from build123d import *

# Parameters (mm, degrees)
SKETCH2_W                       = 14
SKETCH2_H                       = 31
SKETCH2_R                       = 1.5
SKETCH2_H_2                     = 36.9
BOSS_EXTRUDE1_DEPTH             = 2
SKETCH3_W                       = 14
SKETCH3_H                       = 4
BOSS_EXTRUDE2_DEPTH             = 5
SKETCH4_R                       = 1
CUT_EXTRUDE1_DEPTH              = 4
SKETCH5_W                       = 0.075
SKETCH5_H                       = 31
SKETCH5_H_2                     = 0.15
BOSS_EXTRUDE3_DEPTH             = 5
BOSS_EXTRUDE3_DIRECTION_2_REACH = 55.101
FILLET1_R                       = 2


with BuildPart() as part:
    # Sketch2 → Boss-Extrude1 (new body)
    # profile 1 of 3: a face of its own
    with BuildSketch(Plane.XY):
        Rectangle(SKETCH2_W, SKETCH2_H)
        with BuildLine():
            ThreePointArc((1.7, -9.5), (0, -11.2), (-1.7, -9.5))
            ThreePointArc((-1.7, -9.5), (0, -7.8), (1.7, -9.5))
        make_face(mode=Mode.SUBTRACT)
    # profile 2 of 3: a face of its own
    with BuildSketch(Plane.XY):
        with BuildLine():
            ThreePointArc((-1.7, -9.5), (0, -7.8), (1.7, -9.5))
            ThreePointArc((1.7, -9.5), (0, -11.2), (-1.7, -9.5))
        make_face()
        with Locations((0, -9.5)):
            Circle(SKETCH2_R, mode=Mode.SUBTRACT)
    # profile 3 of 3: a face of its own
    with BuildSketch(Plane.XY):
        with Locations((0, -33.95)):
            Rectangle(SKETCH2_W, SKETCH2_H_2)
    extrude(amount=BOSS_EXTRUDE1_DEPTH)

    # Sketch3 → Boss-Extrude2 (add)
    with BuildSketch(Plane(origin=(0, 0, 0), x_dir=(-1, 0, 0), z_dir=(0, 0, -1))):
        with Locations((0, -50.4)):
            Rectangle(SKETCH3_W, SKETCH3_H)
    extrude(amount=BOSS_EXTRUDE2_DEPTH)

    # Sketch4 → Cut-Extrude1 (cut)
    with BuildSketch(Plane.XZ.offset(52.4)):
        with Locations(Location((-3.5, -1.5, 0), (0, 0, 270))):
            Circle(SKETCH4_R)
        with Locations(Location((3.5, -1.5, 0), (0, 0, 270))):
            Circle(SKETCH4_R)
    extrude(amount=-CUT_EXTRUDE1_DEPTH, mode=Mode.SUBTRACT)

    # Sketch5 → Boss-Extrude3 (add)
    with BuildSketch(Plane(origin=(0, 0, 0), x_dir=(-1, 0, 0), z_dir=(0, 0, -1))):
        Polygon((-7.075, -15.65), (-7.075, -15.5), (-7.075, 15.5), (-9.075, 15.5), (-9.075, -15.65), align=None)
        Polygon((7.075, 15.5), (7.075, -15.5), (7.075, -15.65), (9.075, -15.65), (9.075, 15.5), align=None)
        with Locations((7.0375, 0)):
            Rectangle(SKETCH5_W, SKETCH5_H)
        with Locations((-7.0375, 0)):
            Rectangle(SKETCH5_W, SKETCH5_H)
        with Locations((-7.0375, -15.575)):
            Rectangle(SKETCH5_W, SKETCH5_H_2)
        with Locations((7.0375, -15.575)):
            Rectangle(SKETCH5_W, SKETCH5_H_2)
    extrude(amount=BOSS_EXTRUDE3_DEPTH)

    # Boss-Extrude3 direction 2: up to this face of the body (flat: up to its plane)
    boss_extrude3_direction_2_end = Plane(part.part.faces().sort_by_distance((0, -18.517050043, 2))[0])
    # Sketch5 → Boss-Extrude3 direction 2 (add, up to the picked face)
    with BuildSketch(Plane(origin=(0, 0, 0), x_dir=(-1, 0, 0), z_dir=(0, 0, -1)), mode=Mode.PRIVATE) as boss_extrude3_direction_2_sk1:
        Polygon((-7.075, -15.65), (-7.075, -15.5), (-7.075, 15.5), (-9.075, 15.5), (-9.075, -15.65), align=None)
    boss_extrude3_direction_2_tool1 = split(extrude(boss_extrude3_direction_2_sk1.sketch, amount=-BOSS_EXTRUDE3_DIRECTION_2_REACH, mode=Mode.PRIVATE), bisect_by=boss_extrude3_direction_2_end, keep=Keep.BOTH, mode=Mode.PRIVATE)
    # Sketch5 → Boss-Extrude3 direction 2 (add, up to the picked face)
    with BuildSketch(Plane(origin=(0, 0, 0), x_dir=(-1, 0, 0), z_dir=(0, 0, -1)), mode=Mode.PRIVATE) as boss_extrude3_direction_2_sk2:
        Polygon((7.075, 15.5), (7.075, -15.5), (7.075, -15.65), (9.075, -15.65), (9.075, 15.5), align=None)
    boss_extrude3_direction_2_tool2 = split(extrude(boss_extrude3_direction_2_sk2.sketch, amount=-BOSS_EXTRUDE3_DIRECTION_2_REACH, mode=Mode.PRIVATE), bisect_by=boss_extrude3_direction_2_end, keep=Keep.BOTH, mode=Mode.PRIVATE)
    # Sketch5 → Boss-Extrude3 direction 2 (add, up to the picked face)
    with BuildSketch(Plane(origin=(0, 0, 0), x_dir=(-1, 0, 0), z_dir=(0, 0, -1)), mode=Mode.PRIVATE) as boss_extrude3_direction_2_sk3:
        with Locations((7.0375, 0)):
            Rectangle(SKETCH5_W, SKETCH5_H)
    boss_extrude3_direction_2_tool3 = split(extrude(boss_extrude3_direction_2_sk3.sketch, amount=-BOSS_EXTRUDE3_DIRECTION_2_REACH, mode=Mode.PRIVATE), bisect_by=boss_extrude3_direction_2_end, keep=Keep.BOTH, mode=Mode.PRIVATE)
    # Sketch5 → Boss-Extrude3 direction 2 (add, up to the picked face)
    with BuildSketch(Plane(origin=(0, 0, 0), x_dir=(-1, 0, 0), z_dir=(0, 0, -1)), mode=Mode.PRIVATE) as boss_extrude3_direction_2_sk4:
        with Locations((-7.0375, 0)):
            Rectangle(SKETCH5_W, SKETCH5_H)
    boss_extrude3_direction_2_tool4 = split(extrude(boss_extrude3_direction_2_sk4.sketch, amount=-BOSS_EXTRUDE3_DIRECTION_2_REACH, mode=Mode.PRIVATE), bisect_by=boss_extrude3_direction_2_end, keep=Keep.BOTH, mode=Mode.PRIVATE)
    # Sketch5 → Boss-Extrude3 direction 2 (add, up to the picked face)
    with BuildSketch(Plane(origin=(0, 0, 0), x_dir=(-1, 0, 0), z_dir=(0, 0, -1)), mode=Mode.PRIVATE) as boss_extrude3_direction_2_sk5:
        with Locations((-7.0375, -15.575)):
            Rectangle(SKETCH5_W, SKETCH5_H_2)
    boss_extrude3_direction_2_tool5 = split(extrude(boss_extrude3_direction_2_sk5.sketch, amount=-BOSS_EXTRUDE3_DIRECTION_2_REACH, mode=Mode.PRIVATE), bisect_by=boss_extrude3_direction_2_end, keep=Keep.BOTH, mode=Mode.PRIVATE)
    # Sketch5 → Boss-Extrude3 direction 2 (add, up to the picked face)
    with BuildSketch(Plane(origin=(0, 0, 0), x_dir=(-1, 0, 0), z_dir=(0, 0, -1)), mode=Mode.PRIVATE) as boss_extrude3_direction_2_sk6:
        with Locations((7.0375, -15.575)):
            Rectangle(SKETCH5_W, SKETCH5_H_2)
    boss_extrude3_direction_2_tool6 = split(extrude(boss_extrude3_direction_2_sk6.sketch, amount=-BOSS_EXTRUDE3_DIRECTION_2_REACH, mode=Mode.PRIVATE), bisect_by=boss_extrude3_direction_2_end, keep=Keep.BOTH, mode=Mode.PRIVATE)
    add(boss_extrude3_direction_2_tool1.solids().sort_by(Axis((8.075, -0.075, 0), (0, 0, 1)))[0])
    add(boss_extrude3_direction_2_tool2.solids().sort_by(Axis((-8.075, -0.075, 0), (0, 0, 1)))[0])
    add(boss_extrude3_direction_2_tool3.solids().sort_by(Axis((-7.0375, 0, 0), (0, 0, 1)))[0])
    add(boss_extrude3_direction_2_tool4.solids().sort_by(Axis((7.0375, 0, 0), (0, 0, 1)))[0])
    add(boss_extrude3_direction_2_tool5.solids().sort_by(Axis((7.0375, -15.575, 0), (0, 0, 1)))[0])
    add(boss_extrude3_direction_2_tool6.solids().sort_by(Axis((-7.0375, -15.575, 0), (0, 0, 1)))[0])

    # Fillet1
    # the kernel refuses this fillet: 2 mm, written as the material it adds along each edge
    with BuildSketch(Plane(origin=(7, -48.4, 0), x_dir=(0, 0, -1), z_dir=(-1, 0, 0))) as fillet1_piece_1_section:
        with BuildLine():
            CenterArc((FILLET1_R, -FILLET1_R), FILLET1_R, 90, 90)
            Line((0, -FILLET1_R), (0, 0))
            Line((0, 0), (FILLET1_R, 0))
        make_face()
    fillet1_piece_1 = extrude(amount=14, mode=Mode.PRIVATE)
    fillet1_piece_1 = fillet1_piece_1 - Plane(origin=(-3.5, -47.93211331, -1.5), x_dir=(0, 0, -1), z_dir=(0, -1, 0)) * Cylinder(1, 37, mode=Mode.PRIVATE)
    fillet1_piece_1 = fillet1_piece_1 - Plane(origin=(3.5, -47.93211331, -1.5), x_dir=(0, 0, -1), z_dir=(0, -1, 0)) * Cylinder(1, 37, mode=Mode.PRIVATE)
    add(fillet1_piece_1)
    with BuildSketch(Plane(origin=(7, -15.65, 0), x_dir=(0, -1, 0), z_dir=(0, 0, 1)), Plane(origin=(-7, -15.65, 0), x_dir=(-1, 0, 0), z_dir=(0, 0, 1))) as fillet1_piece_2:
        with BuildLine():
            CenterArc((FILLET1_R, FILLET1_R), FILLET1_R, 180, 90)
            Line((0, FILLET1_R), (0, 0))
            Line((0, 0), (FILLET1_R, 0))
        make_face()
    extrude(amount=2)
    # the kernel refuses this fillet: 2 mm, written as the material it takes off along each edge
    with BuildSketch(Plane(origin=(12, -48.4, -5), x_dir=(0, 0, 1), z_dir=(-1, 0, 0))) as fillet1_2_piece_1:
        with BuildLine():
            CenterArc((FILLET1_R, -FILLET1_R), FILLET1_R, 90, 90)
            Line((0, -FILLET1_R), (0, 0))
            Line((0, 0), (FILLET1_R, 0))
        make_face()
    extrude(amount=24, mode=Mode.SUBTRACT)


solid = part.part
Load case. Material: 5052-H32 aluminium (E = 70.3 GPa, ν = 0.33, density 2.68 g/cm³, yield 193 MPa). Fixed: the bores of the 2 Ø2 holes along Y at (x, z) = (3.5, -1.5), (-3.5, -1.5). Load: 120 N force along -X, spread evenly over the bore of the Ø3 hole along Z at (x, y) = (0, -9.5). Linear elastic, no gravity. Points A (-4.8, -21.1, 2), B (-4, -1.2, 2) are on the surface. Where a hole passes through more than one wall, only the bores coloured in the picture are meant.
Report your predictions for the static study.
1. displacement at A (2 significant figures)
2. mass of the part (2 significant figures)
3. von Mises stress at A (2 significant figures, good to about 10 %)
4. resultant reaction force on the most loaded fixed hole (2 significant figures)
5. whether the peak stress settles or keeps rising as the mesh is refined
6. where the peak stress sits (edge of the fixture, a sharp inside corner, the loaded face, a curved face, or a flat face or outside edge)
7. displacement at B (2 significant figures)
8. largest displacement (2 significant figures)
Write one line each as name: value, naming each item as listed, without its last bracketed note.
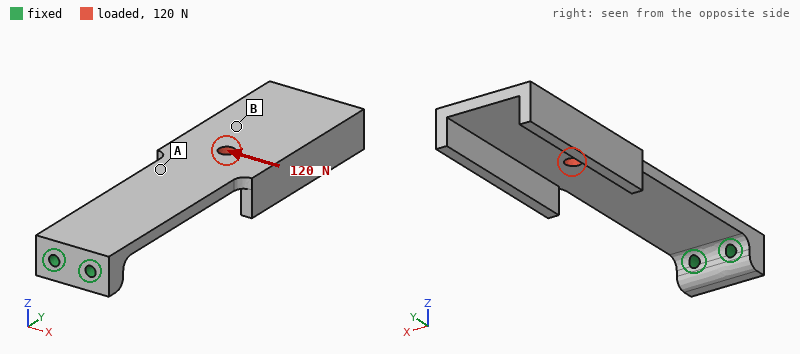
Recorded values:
displacement at A: 0.064 mm
mass of the part: 8.2 g
von Mises stress at A: 16 MPa
resultant reaction force on the most loaded fixed hole: 490 N
whether the peak stress settles or keeps rising as the mesh is refined: keeps rising
where the peak stress sits: edge of the fixture
displacement at B: 0.13 mm
largest displacement: 0.20 mm
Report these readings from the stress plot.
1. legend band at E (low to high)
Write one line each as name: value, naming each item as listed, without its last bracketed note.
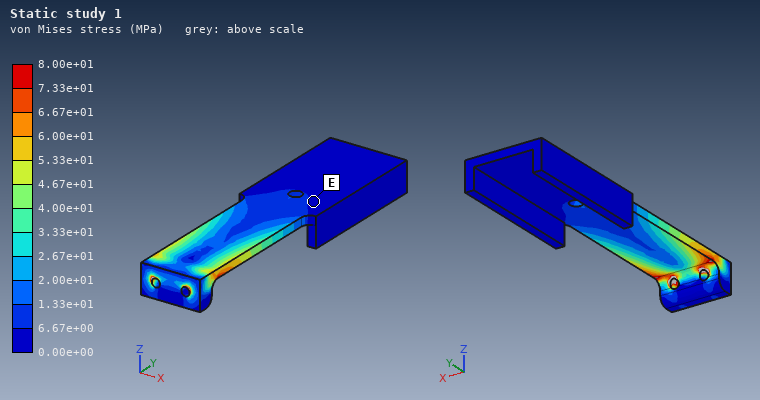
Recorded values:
legend band at E: 0.00e+00 to 6.67e+00 MPa
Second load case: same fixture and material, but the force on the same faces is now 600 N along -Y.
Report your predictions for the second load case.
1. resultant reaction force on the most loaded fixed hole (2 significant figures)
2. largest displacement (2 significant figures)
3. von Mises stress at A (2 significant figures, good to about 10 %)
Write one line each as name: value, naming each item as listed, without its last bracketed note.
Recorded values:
resultant reaction force on the most loaded fixed hole: 300 N
largest displacement: 55 µm
von Mises stress at A: 21 MPa
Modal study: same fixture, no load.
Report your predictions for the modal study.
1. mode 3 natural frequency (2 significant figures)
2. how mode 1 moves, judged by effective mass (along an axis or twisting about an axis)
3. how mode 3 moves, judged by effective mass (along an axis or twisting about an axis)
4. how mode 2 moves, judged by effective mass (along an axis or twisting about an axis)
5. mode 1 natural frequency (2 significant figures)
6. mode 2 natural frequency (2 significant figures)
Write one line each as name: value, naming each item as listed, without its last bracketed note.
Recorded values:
mode 3 natural frequency: 1900 Hz
how mode 1 moves, judged by effective mass: along Z
how mode 3 moves, judged by effective mass: along X
how mode 2 moves, judged by effective mass: along X
mode 1 natural frequency: 300 Hz
mode 2 natural frequency: 1600 Hz
